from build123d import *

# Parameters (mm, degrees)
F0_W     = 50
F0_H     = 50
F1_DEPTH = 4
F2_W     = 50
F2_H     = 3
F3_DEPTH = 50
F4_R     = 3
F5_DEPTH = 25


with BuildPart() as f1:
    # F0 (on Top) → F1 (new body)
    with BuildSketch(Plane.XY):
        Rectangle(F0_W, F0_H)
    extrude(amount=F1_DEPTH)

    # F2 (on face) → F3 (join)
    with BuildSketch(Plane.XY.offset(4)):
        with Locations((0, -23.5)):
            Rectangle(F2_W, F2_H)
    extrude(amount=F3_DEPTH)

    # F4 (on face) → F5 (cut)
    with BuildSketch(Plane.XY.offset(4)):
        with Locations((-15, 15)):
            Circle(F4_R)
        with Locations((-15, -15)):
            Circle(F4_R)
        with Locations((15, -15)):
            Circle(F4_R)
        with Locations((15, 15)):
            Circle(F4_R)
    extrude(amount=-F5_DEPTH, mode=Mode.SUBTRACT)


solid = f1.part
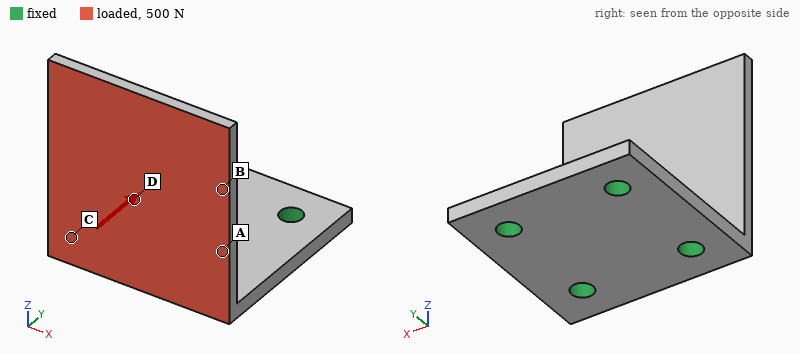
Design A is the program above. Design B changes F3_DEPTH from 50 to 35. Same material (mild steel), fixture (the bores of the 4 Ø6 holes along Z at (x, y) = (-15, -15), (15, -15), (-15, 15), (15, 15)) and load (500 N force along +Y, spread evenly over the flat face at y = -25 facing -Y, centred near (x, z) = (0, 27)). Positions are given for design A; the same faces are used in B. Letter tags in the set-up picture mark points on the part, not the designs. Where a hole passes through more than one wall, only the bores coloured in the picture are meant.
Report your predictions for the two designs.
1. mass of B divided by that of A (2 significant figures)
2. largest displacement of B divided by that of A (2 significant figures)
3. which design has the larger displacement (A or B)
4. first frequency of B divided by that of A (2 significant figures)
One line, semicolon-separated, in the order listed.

0.87; 0.38; A; 1.9
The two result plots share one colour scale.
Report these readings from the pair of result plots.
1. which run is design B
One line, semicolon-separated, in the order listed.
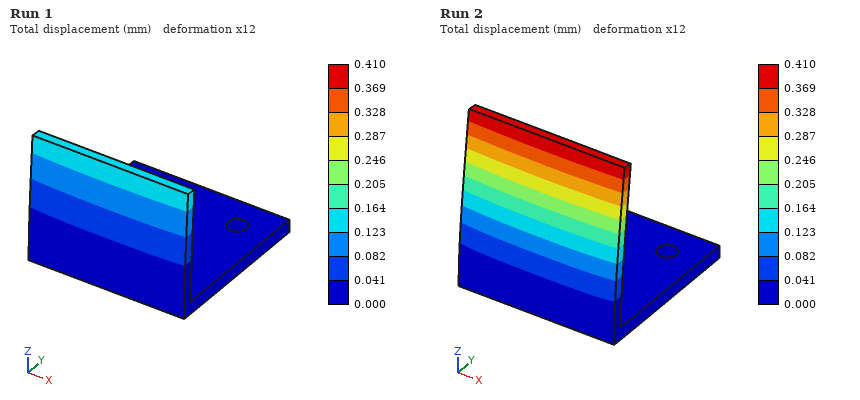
Run 1
